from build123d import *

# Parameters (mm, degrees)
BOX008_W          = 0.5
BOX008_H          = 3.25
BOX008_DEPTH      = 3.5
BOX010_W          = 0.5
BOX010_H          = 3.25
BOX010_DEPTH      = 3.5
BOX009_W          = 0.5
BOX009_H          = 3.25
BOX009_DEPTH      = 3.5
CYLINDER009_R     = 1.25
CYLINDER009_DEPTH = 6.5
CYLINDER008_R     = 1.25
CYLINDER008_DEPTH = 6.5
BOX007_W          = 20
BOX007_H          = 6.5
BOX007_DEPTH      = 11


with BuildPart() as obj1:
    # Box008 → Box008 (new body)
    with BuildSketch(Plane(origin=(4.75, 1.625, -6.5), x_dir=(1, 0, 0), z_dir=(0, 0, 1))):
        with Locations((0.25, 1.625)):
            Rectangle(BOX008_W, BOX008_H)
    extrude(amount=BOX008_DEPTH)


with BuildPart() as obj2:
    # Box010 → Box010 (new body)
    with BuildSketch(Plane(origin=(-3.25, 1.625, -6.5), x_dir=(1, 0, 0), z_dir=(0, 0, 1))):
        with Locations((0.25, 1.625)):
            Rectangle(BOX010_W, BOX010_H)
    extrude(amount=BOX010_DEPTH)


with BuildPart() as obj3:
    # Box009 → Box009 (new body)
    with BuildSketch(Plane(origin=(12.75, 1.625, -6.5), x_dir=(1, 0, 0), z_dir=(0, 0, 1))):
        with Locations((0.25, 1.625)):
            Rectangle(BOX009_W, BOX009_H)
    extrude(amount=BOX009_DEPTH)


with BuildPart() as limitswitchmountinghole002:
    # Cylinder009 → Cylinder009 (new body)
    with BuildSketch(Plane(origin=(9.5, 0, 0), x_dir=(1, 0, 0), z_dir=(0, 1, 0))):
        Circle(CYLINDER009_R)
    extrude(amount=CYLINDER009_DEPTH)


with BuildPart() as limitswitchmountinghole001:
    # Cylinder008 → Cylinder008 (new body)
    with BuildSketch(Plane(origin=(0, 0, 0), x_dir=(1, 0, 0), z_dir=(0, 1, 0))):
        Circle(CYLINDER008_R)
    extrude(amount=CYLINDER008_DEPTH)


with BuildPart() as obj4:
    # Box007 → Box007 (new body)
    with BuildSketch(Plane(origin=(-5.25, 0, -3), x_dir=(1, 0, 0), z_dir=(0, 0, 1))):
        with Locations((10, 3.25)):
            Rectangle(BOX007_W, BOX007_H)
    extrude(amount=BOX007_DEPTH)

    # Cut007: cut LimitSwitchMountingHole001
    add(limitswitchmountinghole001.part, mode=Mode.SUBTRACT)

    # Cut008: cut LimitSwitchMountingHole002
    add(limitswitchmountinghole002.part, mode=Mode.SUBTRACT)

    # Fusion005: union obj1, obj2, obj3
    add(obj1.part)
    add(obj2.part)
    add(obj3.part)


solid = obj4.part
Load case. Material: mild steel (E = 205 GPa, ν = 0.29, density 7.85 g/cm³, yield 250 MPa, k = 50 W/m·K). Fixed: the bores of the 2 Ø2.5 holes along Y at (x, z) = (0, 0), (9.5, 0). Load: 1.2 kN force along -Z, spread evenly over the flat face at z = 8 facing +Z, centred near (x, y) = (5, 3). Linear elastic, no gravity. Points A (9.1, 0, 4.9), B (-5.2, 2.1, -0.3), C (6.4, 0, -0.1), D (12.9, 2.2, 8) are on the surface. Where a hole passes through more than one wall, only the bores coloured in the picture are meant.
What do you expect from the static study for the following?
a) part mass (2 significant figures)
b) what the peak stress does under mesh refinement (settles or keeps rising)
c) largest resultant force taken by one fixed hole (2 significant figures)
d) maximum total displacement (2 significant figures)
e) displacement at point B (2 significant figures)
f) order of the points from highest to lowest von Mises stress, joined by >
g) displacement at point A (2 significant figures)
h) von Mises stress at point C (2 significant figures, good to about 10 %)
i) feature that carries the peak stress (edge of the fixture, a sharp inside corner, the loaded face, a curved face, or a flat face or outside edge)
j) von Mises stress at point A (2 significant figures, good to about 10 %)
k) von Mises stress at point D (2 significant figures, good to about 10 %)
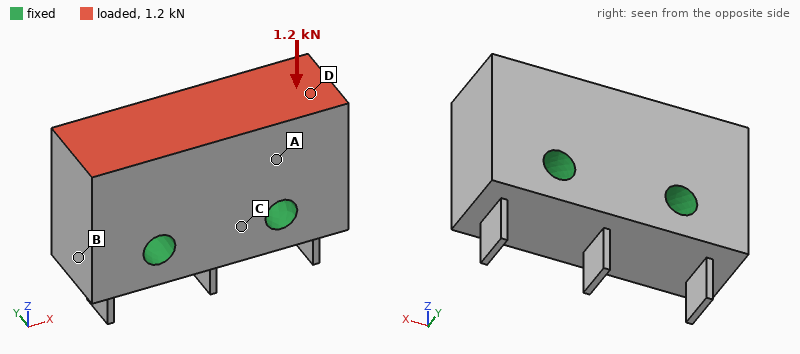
11 g
keeps rising
600 N
0.60 µm
0.31 µm
A > D > C > B
0.27 µm
4.7 MPa
edge of the fixture
11 MPa
9.5 MPa
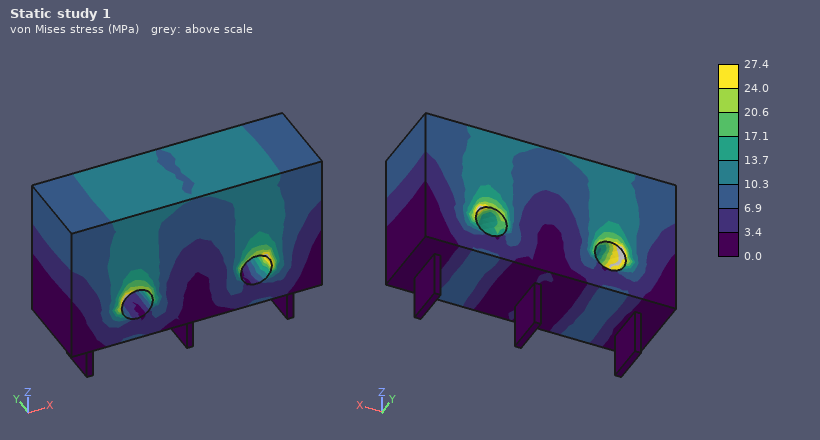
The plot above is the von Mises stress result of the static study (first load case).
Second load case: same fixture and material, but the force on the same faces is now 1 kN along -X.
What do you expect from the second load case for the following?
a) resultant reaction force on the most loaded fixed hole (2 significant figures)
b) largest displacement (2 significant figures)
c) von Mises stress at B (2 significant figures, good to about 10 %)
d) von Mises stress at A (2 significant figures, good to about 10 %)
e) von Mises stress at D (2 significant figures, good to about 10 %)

800 N
2.1 µm
6.1 MPa
17 MPa
19 MPa
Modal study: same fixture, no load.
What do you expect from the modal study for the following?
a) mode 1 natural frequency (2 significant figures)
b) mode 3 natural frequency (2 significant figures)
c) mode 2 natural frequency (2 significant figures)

32 kHz
32 kHz
32 kHz
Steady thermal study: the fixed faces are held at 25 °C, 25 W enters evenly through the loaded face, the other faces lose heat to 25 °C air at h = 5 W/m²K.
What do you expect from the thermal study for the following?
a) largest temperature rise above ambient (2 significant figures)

32 K
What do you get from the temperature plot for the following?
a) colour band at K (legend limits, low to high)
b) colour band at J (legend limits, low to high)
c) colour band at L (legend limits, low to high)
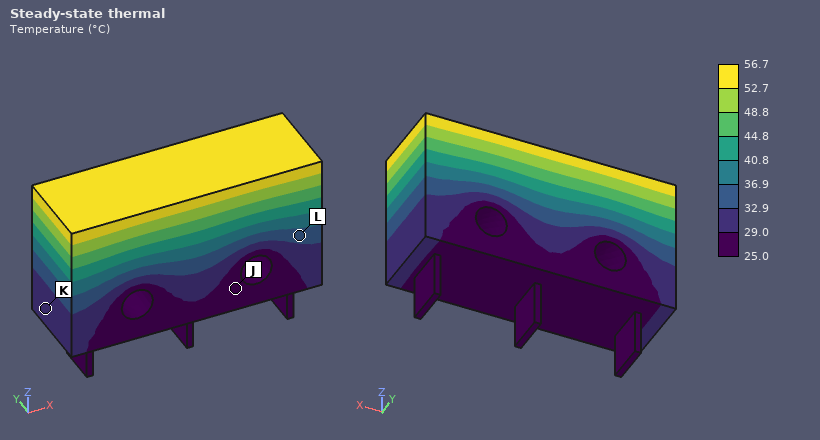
29.0 to 32.9 °C
25.0 to 29.0 °C
32.9 to 36.9 °C
